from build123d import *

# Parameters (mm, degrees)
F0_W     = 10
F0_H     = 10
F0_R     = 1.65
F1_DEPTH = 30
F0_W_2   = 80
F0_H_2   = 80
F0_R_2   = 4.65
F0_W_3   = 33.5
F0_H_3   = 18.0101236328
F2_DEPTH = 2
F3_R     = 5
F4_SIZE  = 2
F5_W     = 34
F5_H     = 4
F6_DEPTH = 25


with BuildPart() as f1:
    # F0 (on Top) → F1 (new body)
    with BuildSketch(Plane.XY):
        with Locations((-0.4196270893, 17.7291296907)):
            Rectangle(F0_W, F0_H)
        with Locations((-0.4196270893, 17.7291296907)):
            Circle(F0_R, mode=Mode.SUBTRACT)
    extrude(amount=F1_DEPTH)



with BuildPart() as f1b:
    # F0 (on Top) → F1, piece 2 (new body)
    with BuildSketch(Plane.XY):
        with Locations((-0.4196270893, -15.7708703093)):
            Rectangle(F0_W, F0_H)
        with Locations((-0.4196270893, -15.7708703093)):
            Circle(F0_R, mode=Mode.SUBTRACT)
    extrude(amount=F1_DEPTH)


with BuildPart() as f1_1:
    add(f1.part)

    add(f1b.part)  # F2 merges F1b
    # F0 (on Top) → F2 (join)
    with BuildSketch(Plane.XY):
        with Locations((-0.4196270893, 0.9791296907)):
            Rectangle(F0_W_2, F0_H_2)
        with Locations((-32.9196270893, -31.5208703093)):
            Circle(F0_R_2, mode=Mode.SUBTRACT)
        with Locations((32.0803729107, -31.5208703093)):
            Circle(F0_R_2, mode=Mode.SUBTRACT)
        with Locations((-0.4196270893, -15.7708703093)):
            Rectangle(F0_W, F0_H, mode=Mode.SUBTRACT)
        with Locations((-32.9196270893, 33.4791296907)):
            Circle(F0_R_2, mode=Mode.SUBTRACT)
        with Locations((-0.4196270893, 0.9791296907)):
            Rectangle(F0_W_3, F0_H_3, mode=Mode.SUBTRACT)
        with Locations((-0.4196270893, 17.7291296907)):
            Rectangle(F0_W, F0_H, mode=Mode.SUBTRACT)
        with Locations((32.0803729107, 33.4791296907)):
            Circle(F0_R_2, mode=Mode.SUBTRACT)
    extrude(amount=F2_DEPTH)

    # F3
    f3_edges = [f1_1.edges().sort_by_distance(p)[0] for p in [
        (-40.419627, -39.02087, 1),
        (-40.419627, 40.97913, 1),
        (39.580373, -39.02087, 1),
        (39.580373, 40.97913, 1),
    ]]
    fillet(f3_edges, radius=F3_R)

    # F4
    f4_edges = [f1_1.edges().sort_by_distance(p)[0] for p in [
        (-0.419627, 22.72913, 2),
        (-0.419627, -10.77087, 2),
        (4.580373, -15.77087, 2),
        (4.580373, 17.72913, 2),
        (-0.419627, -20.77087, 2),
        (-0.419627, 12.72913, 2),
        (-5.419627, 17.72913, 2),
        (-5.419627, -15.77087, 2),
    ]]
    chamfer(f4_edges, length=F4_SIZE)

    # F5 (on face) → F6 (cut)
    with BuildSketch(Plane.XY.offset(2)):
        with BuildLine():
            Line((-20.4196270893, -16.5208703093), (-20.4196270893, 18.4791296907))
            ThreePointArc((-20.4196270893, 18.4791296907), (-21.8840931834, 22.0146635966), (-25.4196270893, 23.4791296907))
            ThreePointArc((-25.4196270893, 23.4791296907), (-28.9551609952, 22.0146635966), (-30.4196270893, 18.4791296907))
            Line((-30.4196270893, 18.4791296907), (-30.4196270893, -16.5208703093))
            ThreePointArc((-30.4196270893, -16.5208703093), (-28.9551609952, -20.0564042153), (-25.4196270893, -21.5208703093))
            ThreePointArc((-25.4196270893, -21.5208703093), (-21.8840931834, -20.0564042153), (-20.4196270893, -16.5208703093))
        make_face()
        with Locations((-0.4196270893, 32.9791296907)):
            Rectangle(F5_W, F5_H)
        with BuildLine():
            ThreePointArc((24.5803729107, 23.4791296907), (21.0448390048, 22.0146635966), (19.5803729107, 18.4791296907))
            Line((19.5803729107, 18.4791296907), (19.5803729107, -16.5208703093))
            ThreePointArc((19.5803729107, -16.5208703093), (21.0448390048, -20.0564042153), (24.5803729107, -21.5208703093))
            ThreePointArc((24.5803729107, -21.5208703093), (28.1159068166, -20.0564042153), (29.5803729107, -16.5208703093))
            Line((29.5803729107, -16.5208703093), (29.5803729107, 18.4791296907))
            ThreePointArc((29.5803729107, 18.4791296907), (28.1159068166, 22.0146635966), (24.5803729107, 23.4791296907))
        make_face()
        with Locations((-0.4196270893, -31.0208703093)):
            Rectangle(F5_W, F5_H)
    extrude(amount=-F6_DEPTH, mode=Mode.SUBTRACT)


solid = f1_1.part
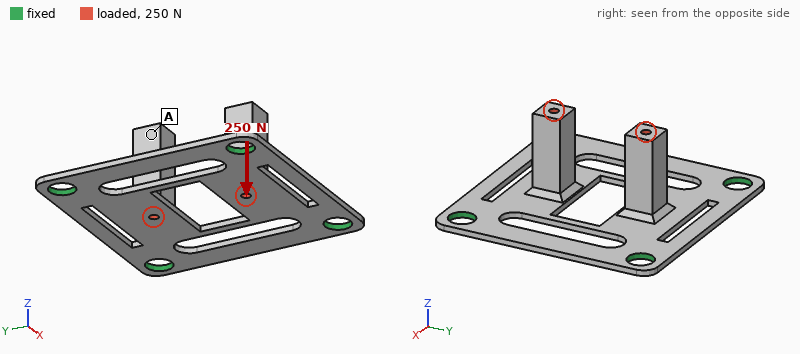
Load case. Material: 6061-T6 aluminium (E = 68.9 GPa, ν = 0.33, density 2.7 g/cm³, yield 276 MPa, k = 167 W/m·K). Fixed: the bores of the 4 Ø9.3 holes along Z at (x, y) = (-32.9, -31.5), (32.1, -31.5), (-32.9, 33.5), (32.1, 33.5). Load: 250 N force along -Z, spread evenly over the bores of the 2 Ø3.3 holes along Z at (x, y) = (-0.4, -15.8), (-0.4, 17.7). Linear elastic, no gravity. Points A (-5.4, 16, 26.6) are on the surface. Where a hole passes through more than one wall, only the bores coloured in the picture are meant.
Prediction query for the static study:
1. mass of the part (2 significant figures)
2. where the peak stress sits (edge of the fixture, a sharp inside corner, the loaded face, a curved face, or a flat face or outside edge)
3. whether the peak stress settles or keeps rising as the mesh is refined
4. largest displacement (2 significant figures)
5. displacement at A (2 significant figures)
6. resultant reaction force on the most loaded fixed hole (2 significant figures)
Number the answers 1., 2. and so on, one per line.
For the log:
1. 38 g
2. edge of the fixture
3. keeps rising
4. 0.39 mm
5. 0.34 mm
6. 65 N
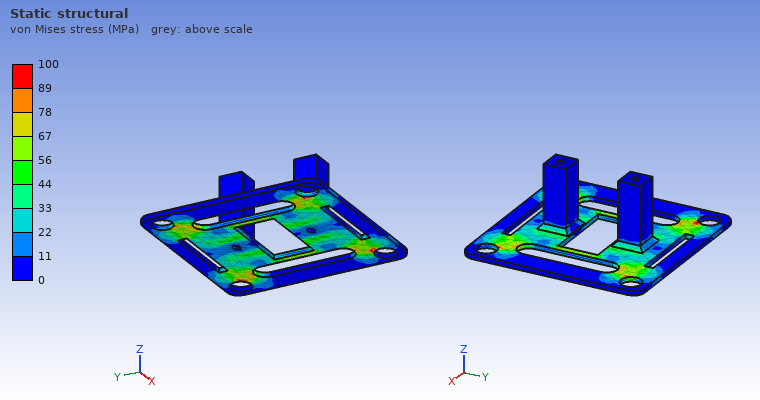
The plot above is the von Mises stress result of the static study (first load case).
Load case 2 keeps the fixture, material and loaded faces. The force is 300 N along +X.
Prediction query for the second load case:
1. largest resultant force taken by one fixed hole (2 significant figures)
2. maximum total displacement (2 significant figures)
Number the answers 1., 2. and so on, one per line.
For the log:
1. 96 N
2. 0.15 mm
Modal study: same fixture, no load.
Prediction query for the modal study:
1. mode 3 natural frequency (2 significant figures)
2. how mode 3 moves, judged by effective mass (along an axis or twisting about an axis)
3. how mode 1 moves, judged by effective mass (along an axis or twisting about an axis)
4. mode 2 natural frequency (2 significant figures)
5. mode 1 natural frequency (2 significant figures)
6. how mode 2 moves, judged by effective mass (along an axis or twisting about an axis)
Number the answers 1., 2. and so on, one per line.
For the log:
1. 2000 Hz
2. along Z
3. along Z
4. 1500 Hz
5. 890 Hz
6. along Y
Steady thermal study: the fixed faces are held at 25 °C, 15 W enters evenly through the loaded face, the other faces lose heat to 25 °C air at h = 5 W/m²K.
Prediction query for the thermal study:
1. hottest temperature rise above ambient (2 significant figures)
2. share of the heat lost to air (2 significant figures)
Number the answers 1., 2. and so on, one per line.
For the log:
1. 27 K
2. 4.4 %
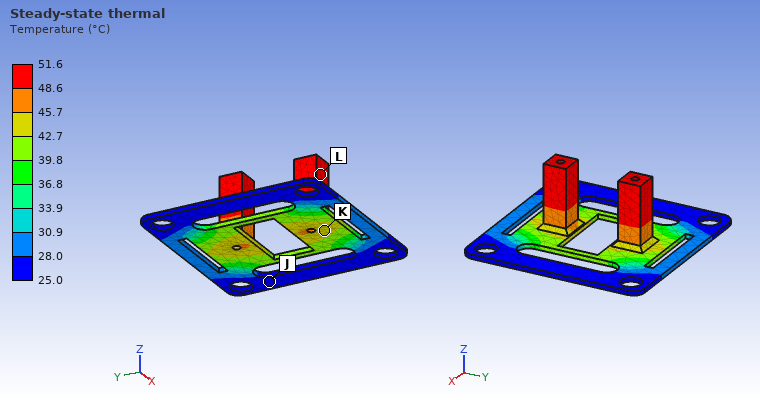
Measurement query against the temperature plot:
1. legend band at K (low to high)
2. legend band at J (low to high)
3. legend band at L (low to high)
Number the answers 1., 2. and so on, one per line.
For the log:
1. 42.7 to 45.7 °C
2. 25.0 to 28.0 °C
3. 48.6 to 51.6 °C
